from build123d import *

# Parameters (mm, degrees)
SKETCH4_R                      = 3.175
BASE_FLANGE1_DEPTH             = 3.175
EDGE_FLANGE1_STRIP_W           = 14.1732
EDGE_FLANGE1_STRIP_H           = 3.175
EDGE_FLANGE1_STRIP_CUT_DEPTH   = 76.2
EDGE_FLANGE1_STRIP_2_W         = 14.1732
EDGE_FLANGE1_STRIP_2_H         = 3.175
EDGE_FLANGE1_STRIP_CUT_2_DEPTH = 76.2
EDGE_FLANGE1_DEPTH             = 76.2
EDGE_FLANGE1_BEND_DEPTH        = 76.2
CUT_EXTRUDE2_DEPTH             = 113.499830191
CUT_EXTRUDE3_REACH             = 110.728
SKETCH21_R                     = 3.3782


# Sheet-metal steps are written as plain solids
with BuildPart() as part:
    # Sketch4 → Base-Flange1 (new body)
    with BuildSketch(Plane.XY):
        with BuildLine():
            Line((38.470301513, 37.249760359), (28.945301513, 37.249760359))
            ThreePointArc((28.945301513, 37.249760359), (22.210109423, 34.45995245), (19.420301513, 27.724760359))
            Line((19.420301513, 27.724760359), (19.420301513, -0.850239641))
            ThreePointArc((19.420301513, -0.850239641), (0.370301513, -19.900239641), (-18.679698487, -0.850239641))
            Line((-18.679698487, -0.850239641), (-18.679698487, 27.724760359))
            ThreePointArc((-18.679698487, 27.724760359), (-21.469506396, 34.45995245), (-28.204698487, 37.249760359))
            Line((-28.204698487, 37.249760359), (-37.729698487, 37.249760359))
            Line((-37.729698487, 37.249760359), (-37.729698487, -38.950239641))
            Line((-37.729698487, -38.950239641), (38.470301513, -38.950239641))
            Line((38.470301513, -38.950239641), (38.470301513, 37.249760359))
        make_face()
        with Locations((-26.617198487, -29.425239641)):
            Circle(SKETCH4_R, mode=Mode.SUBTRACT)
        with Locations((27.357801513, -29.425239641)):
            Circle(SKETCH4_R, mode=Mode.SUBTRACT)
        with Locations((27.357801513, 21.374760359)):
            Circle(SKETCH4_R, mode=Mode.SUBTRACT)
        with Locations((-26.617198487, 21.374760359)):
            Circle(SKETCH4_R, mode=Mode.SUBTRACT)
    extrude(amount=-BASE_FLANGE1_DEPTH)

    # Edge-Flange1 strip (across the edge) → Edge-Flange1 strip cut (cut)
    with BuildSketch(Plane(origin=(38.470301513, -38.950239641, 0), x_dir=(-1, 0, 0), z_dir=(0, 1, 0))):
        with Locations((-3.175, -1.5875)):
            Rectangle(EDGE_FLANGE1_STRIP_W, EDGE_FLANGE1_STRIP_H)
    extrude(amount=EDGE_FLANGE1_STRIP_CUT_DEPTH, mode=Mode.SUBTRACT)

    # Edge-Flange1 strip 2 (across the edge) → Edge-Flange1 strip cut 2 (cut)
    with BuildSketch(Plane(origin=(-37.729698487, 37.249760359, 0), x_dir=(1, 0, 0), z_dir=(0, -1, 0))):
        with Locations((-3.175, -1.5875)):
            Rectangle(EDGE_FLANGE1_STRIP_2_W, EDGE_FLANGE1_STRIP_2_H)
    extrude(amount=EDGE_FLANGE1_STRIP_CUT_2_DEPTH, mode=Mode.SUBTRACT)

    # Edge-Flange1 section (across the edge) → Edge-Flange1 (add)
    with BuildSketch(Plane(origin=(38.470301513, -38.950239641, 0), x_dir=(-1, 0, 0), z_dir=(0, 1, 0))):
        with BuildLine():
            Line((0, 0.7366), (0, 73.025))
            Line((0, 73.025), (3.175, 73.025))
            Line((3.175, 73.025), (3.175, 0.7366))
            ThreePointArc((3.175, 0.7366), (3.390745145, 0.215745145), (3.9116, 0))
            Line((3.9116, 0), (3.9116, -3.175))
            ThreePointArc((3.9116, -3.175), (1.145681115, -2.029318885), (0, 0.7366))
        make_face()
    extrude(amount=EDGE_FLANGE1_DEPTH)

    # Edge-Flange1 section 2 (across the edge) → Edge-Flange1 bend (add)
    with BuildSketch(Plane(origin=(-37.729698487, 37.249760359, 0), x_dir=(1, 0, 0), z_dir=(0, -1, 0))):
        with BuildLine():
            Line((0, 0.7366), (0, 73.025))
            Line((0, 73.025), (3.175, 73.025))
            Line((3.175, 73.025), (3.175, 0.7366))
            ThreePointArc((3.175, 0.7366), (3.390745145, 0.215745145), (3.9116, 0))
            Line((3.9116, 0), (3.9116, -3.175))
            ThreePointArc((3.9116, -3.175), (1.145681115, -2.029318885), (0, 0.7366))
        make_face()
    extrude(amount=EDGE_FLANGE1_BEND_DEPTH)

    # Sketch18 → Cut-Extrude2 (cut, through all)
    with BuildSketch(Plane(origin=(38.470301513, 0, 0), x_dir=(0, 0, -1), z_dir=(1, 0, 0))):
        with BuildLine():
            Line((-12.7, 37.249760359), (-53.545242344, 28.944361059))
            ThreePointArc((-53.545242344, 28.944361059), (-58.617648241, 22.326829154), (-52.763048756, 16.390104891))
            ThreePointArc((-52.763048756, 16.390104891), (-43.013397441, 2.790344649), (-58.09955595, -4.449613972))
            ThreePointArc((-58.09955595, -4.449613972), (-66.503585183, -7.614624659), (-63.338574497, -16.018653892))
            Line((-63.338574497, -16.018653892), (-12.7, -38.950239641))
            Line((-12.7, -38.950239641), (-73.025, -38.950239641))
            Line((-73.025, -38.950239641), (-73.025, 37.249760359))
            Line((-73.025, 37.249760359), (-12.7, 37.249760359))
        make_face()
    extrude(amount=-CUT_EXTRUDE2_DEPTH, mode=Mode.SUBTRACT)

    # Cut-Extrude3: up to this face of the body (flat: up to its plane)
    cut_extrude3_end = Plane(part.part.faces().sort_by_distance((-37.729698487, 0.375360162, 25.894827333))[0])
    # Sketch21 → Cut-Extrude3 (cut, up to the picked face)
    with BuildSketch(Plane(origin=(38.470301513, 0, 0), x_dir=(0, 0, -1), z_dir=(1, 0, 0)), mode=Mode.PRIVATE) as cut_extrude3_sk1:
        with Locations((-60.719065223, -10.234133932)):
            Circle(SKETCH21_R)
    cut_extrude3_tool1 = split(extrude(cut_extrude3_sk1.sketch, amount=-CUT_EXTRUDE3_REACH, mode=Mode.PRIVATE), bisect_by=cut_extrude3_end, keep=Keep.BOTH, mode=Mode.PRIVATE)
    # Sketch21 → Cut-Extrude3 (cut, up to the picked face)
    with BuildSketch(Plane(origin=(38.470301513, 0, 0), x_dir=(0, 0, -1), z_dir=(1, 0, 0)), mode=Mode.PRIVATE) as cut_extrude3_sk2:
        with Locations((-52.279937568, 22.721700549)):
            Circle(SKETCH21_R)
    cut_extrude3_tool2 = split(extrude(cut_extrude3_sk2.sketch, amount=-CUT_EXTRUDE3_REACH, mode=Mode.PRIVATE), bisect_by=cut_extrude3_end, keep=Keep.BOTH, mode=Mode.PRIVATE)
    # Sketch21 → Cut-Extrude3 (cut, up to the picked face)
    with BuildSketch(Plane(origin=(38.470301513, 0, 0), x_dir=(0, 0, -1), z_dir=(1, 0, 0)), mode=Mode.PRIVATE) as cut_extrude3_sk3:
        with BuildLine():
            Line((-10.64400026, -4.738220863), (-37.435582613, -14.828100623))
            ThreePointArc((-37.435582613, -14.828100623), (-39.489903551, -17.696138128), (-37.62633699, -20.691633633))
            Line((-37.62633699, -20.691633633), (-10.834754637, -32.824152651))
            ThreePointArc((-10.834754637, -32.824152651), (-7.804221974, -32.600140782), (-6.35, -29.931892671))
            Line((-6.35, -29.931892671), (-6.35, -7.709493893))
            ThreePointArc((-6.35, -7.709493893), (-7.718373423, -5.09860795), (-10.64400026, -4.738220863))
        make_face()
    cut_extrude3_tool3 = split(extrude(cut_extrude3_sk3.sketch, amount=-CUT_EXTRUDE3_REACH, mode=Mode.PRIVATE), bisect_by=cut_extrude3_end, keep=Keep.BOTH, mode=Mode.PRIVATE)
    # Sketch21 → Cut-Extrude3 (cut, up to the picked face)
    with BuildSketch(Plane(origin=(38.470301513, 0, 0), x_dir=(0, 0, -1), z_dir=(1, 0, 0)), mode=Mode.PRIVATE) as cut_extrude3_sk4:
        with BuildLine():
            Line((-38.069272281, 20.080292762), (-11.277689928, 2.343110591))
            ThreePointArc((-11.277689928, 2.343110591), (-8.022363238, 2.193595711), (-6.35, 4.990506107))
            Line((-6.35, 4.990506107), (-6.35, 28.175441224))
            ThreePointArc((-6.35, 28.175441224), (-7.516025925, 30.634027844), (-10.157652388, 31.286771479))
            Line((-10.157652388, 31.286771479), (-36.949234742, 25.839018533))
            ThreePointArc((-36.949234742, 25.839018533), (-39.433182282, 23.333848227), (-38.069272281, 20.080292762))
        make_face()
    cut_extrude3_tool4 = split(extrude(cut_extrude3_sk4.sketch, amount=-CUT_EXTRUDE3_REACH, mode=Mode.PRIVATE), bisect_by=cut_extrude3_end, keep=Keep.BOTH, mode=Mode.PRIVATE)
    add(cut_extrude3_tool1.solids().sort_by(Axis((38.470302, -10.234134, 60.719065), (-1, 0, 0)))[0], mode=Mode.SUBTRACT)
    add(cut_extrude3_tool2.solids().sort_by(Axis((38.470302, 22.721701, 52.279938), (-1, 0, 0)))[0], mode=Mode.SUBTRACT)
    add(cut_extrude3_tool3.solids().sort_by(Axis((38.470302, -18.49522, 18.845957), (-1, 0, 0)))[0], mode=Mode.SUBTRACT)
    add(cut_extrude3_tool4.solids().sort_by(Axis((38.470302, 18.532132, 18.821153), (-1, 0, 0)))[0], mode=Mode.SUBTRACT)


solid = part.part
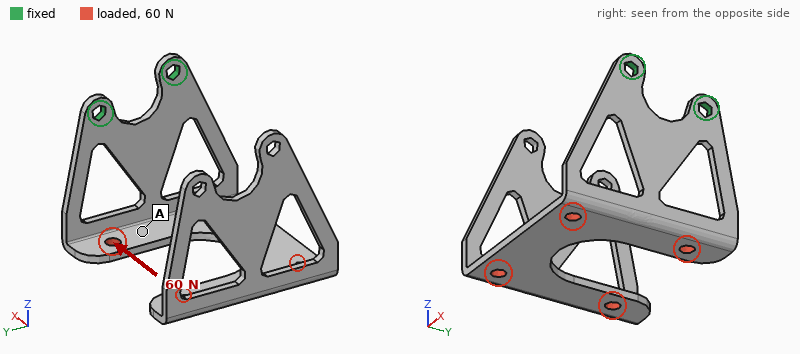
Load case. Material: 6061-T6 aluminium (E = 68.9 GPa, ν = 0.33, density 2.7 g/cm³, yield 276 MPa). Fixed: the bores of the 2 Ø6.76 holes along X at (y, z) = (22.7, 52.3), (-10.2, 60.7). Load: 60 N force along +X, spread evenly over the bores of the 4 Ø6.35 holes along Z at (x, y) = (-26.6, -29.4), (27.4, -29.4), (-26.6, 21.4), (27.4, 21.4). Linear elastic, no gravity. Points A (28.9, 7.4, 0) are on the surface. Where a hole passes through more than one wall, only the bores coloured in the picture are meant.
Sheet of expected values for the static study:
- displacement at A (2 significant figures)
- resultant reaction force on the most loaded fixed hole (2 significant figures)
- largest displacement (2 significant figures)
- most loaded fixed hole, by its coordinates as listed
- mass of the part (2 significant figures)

0.54 mm
33 N
1.4 mm
(22.7, 52.3)
69 g
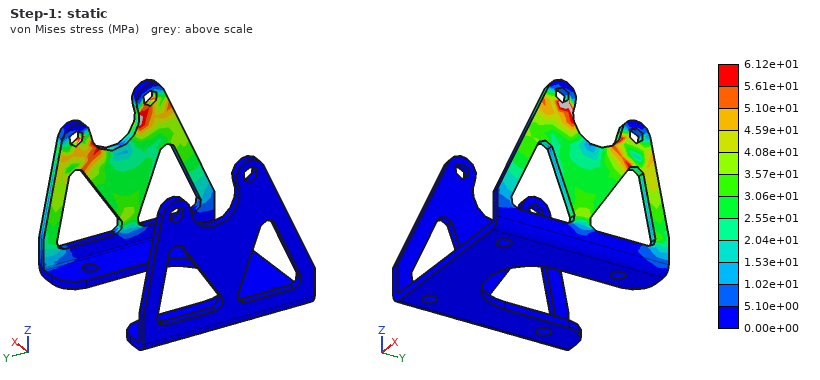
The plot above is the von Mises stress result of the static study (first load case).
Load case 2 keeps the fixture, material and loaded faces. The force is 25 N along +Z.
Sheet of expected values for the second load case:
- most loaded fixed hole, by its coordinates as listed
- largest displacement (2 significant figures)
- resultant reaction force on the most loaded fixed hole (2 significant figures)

(-10.2, 60.7)
1.3 mm
20 N
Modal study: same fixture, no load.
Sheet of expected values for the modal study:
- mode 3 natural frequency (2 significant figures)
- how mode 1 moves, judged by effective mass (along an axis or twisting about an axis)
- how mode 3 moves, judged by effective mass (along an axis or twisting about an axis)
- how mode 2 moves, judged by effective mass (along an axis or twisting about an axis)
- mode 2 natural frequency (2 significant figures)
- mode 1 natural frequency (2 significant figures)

240 Hz
along Z
along X
along Y
160 Hz
91 Hz
